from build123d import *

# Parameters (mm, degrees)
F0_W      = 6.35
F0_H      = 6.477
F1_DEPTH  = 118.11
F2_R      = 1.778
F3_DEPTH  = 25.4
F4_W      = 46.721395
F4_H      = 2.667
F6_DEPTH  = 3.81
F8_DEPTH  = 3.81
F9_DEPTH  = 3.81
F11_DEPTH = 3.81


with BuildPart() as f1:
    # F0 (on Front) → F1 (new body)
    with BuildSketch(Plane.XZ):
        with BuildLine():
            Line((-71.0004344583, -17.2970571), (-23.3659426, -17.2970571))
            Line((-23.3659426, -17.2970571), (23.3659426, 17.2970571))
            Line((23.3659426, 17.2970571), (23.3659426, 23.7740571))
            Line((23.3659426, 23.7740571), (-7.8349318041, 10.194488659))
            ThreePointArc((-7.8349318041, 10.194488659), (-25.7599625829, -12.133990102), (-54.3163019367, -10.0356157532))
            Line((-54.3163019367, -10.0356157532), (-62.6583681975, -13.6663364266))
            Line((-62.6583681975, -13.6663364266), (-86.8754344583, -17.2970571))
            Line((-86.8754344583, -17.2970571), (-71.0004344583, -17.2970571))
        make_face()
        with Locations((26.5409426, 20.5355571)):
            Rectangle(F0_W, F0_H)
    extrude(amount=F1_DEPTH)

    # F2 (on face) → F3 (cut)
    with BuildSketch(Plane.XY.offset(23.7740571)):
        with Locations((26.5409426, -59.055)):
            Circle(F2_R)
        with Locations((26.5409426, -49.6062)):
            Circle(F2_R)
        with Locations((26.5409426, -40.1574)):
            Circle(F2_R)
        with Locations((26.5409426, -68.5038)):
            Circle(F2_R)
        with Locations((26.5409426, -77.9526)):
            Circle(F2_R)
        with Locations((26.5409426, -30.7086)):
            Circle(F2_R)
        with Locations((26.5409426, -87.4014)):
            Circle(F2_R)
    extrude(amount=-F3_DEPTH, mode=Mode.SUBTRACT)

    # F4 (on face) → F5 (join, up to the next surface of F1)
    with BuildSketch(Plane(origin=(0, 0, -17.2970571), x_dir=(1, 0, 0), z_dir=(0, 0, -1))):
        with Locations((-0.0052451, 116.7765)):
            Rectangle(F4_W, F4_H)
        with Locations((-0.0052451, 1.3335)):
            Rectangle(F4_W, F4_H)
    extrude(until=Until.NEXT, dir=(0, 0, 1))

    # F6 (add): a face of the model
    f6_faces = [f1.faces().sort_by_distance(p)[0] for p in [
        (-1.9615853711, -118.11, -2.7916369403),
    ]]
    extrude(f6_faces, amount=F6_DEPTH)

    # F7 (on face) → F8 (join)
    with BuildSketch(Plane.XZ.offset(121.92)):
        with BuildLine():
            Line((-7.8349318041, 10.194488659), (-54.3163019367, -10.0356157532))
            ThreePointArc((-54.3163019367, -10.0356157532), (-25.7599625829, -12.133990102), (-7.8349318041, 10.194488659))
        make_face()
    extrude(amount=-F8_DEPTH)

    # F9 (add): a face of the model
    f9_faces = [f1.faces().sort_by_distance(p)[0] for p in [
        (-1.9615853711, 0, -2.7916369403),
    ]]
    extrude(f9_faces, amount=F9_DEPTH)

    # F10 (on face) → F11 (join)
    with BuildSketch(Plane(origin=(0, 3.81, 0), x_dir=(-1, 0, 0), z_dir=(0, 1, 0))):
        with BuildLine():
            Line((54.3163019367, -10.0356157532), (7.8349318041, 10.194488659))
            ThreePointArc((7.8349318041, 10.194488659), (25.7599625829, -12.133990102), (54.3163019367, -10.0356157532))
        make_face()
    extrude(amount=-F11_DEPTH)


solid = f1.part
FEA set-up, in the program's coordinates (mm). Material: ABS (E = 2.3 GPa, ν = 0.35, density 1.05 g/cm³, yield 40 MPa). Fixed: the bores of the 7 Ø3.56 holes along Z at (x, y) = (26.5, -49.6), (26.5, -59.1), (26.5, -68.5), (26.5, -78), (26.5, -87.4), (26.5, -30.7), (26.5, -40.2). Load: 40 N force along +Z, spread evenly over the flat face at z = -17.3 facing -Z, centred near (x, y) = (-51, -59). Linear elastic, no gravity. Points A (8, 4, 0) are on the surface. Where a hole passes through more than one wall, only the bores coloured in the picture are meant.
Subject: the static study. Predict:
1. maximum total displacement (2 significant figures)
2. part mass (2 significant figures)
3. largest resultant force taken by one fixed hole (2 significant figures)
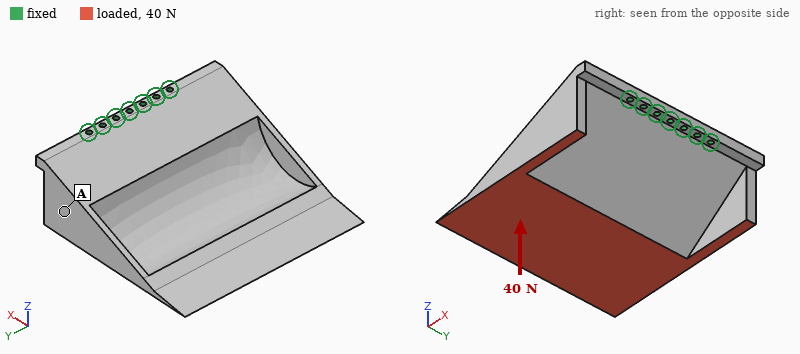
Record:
1.8 mm
110 g
15 N
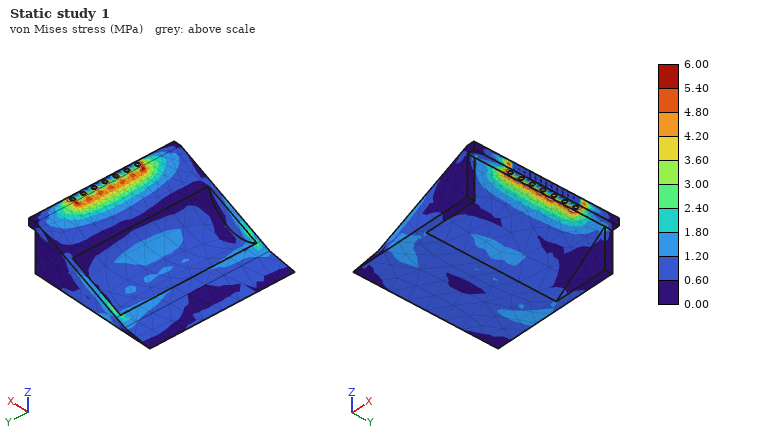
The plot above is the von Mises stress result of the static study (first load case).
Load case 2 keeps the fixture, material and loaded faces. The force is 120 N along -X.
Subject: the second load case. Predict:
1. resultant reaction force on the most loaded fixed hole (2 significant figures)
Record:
39 N
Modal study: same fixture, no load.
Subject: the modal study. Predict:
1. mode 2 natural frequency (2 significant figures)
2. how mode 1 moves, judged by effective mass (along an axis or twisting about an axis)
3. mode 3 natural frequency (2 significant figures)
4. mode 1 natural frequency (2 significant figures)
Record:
280 Hz
along Z
550 Hz
170 Hz
